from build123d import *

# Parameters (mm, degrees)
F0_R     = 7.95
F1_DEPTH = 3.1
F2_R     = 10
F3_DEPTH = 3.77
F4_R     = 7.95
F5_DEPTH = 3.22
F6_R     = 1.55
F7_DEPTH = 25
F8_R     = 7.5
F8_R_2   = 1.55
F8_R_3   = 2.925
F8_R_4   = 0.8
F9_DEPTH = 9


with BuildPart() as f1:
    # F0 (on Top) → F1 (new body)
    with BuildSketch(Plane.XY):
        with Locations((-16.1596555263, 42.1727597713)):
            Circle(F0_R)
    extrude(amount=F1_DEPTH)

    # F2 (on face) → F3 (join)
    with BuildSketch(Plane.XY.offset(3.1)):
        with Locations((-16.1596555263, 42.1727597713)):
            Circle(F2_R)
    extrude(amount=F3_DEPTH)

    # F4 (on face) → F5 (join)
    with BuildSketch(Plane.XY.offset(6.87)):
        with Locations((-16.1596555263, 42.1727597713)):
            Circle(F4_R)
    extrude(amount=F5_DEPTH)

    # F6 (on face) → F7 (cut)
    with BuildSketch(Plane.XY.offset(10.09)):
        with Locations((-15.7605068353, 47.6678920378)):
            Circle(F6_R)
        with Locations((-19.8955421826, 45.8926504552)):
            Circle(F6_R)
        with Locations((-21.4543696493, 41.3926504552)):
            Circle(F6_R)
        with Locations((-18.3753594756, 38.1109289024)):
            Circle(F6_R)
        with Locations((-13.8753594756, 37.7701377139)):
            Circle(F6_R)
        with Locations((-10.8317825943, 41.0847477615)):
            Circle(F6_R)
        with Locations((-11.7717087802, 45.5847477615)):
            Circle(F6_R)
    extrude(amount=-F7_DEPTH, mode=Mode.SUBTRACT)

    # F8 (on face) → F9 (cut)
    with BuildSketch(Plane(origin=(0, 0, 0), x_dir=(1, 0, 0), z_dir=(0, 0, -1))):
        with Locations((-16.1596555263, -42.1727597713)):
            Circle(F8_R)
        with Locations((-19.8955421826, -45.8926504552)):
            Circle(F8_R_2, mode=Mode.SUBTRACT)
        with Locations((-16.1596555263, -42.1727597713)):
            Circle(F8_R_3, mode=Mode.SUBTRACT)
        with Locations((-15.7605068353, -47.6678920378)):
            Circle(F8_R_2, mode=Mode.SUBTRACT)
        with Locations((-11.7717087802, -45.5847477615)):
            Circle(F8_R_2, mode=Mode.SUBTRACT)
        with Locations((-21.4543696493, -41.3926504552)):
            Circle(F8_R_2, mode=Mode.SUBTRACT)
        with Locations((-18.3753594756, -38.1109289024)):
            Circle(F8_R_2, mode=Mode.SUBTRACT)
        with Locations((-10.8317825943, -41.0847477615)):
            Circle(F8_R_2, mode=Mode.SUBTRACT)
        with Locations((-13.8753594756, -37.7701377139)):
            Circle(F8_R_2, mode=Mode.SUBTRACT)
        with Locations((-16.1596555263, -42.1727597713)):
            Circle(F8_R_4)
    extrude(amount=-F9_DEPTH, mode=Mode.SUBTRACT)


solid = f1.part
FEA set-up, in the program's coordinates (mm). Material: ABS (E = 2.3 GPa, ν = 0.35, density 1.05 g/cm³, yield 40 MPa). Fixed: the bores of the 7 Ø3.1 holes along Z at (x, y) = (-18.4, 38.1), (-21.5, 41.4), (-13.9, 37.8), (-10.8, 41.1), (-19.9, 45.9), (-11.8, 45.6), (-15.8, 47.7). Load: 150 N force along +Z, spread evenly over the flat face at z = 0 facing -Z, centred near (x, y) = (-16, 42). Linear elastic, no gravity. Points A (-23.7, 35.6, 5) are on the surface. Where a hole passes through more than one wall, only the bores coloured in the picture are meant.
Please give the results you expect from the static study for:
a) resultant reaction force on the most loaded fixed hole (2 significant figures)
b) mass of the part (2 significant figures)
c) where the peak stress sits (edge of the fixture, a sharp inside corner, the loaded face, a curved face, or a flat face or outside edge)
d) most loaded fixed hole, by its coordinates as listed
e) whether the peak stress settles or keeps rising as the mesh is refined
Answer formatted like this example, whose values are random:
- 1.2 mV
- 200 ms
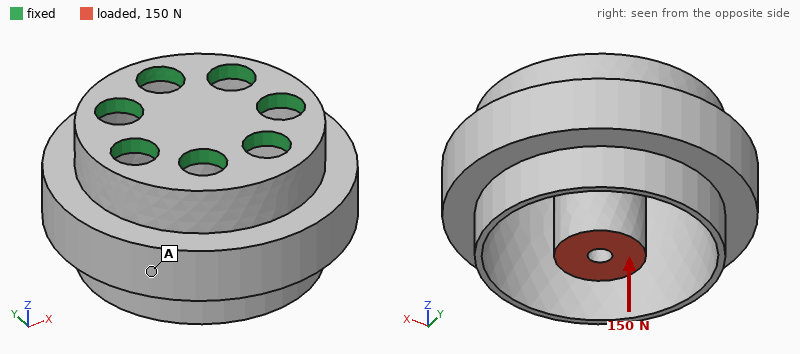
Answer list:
- 36 N
- 1.1 g
- edge of the fixture
- (-18.4, 38.1)
- keeps rising
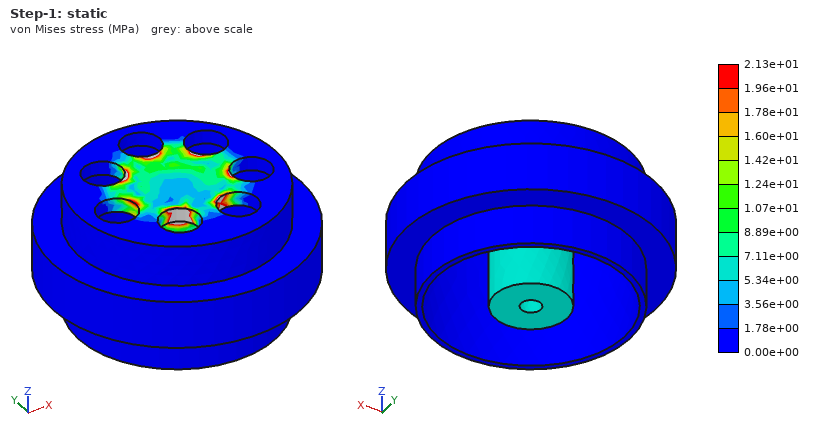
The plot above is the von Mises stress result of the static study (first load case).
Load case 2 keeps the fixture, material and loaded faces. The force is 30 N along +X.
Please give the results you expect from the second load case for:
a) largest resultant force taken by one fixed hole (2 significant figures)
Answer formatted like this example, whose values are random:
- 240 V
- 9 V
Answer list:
- 22 N
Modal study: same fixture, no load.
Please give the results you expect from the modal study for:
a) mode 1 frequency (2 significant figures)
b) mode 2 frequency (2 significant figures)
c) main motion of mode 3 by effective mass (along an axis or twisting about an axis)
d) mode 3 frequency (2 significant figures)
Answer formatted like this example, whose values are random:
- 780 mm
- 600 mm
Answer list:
- 7200 Hz
- 7500 Hz
- along Y
- 8200 Hz
